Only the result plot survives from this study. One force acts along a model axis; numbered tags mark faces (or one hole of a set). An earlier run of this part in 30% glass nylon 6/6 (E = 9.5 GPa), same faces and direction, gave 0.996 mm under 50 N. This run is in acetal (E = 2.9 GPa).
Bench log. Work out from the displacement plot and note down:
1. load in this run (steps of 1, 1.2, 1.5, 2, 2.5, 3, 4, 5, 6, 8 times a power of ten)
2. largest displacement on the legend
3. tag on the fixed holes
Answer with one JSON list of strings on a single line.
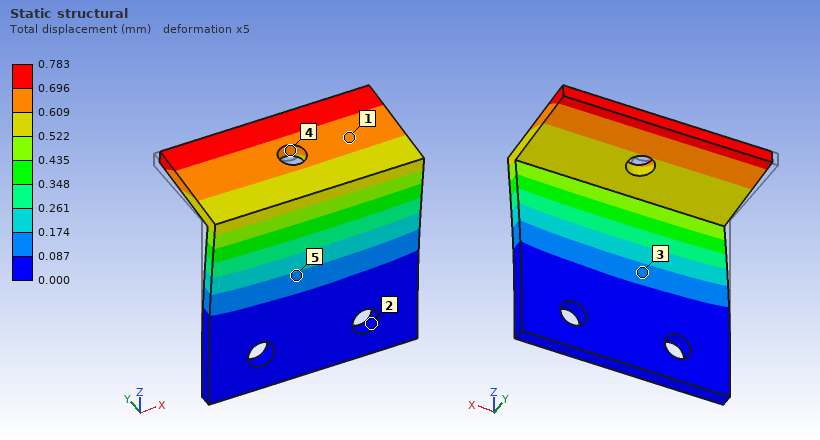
["12 N", "0.783 mm", "2"]
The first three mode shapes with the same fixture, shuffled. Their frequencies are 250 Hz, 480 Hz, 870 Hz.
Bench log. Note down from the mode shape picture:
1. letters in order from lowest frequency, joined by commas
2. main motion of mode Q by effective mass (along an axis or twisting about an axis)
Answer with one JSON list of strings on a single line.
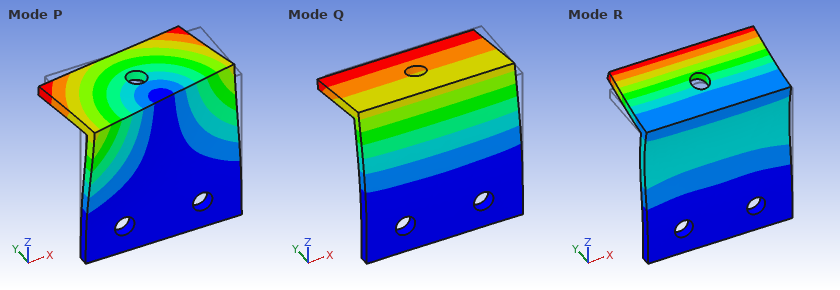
["Q, P, R", "along Y"]
